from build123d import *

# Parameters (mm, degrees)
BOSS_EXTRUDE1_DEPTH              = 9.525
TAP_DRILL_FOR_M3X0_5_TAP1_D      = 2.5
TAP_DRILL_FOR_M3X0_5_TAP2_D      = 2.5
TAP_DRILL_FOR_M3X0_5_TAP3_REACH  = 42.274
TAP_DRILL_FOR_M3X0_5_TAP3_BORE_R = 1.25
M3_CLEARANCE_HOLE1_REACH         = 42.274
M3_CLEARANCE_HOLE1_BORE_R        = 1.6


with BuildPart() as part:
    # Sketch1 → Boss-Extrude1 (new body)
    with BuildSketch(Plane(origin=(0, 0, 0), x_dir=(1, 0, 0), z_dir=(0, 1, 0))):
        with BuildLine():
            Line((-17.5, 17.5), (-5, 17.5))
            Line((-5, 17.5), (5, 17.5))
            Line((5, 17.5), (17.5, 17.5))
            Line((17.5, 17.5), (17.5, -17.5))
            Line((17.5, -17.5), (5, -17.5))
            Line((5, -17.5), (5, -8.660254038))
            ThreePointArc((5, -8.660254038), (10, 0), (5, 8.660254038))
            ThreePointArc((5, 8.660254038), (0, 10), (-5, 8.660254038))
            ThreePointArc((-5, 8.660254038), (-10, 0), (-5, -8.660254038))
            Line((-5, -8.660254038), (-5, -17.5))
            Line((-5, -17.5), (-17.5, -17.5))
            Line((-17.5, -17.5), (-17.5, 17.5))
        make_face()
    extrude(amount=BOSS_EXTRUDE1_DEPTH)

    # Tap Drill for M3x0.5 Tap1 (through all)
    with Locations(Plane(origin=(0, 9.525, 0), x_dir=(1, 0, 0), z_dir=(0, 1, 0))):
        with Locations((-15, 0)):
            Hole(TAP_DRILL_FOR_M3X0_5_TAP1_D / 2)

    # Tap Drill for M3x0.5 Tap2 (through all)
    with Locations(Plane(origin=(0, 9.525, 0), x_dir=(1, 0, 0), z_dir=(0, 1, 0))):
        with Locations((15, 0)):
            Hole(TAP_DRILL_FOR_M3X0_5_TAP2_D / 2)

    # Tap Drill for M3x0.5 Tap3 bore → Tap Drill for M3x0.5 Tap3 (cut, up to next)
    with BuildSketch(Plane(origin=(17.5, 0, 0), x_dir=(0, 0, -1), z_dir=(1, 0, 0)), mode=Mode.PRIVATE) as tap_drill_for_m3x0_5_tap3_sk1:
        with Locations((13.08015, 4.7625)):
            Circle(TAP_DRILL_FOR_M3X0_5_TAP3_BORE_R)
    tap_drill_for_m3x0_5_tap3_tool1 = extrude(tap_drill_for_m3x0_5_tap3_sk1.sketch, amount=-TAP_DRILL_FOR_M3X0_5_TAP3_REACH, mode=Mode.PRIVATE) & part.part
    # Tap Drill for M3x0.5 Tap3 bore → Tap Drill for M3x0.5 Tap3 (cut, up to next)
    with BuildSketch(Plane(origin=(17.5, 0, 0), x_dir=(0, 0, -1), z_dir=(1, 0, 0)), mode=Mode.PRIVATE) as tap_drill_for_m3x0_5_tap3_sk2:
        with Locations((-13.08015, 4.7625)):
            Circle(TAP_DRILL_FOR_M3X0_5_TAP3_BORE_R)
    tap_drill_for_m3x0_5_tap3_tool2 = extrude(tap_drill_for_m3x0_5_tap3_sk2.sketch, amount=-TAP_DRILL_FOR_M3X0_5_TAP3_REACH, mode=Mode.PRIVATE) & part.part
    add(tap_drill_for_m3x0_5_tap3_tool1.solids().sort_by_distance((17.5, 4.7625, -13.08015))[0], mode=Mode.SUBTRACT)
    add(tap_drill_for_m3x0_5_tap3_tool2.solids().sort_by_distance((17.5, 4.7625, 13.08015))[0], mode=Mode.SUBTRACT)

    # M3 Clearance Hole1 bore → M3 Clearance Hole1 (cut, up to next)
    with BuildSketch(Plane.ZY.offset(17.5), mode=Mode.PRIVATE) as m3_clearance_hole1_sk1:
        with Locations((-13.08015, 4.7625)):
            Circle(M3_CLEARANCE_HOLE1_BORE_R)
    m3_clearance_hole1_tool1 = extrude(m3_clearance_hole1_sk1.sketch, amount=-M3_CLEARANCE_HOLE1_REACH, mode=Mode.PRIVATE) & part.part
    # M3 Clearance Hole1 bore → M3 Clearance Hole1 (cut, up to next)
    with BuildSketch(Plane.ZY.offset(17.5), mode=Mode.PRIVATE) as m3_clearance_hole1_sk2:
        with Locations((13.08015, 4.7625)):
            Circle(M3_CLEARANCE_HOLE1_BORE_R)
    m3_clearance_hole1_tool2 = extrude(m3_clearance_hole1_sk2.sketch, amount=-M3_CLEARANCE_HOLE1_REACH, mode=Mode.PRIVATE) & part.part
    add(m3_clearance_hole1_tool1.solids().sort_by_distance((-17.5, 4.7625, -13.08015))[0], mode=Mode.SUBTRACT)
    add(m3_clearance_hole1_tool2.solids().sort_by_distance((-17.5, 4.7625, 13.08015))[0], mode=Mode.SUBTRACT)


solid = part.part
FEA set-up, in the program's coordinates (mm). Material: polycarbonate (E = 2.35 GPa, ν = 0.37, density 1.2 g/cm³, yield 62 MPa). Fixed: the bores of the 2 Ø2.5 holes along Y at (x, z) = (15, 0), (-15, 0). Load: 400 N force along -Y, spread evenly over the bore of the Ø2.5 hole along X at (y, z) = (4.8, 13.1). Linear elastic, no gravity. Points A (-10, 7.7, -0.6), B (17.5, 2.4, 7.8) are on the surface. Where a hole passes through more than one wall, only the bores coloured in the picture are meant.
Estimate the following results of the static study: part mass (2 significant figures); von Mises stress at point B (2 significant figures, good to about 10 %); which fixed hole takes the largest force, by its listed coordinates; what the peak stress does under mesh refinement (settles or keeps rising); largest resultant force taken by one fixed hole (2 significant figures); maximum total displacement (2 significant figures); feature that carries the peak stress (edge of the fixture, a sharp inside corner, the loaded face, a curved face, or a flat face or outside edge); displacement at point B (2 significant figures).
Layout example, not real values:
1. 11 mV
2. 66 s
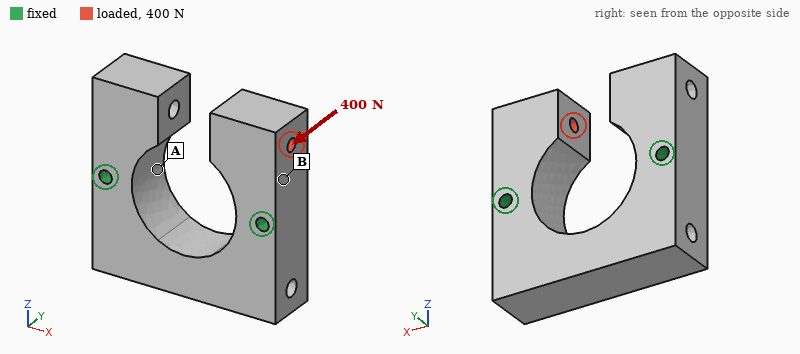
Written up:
1. 8.9 g
2. 11 MPa
3. (15, 0)
4. keeps rising
5. 400 N
6. 0.50 mm
7. edge of the fixture
8. 0.13 mm
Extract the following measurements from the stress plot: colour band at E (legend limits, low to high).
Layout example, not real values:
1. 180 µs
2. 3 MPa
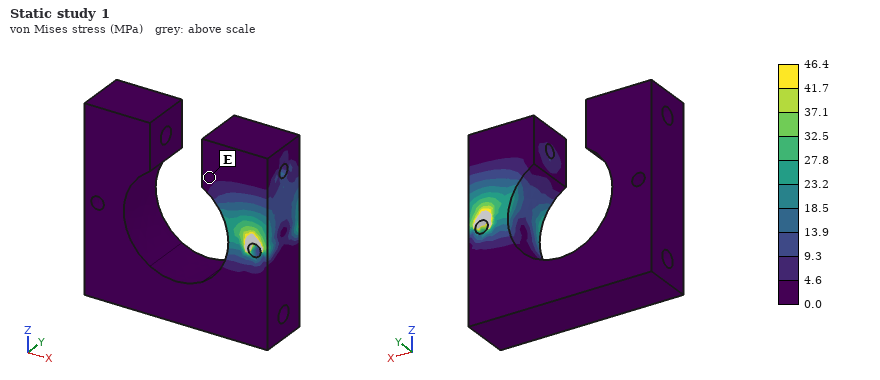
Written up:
1. 0.0 to 4.6 MPa
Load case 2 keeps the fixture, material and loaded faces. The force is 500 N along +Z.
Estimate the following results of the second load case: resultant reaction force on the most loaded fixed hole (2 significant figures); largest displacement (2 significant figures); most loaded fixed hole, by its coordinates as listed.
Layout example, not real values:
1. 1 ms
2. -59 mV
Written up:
1. 480 N
2. 0.30 mm
3. (15, 0)
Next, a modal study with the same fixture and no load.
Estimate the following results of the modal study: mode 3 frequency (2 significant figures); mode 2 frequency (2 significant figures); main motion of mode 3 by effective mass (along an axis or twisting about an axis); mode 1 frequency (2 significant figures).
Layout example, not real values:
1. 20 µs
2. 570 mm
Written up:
1. 3900 Hz
2. 3400 Hz
3. along Y
4. 3300 Hz
